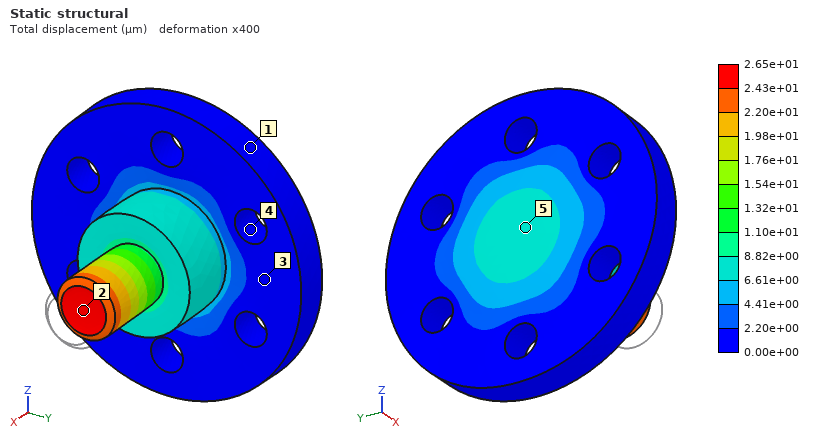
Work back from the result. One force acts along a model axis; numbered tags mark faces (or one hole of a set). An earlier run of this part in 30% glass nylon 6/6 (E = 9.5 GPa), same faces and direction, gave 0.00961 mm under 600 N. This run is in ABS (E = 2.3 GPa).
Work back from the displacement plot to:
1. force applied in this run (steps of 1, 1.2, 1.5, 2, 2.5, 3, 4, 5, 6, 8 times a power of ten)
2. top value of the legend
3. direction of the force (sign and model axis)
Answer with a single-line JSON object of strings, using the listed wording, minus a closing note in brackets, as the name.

{"force applied in this run": "400 N", "top value of the legend": "2.65e+01 µm", "direction of the force": "-X"}
